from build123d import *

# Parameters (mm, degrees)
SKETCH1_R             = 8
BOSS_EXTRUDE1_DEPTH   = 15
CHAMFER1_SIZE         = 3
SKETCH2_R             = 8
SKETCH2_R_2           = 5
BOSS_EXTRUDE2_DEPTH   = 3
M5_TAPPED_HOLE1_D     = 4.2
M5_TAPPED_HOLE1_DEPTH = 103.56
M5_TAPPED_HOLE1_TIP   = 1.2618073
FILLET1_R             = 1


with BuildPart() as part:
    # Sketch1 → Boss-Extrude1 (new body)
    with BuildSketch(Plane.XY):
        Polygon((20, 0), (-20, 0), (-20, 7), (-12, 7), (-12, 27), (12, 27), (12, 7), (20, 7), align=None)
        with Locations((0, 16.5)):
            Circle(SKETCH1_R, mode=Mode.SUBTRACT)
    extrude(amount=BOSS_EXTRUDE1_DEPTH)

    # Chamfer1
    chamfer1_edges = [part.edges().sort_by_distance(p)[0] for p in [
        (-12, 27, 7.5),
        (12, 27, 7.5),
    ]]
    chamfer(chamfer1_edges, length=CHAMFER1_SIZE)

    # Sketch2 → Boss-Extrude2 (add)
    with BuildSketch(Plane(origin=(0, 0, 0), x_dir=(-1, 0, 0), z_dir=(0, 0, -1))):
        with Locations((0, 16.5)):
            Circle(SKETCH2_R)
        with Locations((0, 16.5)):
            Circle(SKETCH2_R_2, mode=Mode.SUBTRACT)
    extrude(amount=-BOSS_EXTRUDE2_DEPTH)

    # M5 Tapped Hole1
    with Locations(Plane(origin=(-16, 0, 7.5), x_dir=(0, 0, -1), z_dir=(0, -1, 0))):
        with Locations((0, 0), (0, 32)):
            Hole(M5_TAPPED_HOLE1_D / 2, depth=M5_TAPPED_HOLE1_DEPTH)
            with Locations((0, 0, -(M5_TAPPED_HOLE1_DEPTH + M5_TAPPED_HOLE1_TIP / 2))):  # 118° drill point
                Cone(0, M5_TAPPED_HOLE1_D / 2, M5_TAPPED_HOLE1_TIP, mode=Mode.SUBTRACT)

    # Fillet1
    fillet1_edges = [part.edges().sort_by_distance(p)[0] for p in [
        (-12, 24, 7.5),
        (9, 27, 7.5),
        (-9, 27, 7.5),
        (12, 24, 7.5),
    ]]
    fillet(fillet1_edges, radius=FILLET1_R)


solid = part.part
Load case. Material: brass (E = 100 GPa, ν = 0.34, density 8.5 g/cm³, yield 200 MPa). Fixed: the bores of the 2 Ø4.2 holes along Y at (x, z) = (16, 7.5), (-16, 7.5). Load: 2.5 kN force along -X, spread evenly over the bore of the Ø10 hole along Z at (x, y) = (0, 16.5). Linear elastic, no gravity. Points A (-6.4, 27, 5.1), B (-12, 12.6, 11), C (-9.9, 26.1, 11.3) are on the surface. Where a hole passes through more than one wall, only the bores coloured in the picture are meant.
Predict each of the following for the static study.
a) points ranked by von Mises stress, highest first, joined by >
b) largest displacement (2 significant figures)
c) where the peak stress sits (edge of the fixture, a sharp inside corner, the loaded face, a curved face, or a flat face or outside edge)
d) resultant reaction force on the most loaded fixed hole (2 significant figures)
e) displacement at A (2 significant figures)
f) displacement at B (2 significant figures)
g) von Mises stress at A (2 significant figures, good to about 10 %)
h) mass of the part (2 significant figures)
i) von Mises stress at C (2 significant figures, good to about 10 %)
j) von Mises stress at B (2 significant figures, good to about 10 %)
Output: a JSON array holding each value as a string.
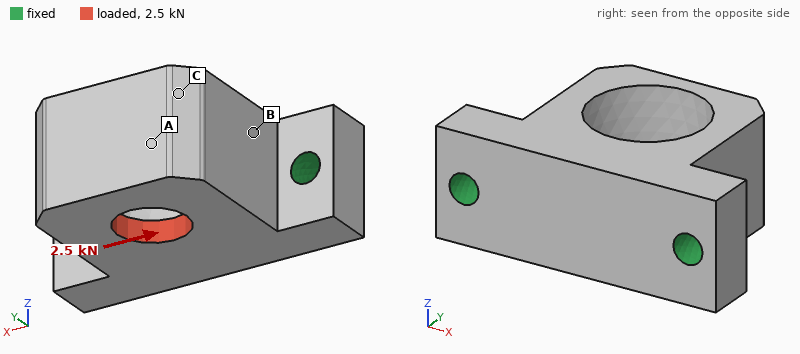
["B > A > C", "21 µm", "the loaded face", "1.8 kN", "18 µm", "6.1 µm", "17 MPa", "72 g", "7.9 MPa", "30 MPa"]
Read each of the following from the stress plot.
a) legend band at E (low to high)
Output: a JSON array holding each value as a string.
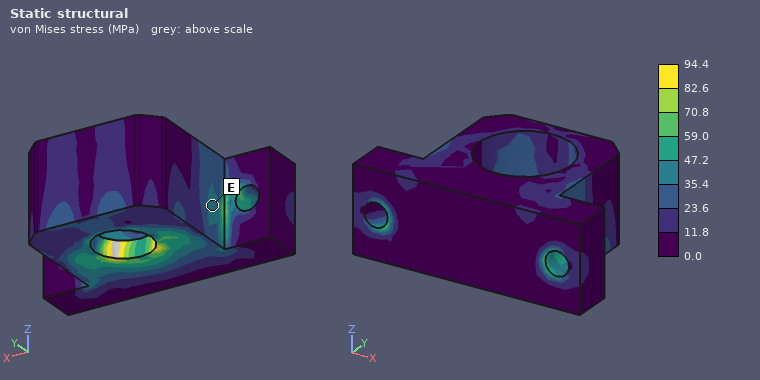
["35.4 to 47.2 MPa"]
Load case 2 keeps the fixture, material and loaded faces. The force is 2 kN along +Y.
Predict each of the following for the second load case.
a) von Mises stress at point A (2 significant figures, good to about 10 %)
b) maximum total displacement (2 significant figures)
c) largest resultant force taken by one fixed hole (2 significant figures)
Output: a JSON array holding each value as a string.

["11 MPa", "25 µm", "1.1 kN"]
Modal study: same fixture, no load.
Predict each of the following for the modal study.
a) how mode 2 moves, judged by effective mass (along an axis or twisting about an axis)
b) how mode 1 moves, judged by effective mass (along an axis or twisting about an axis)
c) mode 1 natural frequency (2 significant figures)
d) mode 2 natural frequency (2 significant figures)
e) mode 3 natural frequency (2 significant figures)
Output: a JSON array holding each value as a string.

["along X", "along Z", "5800 Hz", "9800 Hz", "15 kHz"]
